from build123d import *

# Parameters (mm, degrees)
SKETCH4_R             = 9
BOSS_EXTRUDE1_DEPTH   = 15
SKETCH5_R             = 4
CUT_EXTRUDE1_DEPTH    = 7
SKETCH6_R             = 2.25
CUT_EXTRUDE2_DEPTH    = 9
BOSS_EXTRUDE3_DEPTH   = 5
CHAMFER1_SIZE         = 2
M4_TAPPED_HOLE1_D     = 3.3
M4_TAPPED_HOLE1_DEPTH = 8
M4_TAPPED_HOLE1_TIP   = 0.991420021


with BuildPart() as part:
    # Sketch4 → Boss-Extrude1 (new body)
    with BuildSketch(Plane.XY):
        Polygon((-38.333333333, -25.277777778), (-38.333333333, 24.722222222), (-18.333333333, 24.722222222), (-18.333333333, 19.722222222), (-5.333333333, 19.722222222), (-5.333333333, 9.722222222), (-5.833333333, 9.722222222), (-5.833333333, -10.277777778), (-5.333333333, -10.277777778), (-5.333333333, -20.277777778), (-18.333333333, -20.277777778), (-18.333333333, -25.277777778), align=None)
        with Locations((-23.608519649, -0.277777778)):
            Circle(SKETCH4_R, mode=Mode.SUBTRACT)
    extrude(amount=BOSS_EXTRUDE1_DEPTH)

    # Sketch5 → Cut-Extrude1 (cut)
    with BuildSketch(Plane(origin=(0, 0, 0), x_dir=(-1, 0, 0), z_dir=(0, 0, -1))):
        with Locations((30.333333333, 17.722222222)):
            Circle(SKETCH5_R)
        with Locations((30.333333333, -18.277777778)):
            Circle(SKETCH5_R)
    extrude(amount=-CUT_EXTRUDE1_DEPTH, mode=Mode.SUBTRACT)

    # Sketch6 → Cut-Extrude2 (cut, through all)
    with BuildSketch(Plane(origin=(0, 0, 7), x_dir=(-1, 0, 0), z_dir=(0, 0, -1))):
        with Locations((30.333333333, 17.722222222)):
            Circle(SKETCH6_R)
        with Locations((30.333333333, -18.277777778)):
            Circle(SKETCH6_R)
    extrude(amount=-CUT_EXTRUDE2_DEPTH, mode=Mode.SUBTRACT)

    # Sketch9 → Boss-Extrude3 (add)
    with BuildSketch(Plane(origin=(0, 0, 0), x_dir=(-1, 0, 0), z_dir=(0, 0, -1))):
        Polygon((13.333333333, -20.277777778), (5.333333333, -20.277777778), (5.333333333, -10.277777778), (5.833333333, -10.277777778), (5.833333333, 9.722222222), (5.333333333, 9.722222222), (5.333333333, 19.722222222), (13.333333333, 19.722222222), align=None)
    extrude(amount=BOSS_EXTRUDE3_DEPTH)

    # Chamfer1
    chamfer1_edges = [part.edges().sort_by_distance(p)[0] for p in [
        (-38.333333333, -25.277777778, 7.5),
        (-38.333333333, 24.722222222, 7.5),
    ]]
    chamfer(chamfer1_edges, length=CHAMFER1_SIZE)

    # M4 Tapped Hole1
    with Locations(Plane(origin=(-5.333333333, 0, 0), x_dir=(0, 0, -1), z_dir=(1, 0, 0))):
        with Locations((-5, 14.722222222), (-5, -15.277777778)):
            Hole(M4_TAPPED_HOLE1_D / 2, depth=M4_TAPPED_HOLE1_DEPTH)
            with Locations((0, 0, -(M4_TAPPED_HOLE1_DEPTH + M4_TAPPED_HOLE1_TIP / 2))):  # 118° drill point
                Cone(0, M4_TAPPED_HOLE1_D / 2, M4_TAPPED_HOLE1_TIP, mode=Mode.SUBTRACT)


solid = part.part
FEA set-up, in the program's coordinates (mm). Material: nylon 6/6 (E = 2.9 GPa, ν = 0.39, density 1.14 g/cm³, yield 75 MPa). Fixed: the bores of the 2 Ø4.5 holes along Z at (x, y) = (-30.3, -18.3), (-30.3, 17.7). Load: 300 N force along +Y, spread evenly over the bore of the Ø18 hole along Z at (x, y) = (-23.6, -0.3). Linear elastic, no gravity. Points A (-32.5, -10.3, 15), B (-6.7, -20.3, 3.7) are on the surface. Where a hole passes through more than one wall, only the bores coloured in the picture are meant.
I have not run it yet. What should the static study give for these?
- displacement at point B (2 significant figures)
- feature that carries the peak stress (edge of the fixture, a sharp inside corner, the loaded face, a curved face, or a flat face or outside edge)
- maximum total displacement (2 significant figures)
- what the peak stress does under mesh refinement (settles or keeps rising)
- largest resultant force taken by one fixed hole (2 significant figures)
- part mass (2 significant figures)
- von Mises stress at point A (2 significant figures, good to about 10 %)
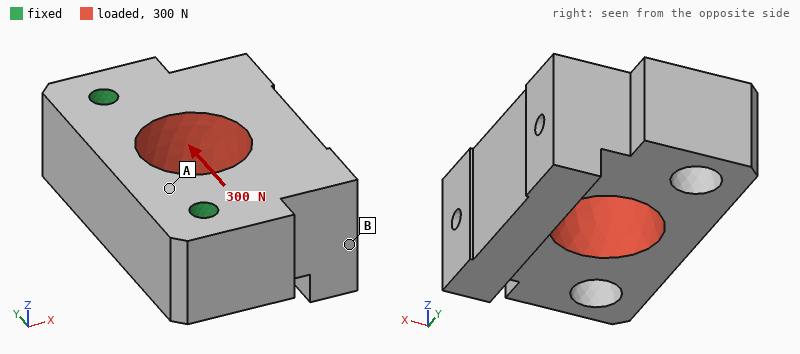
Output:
13 µm
edge of the fixture
14 µm
keeps rising
160 N
22 g
0.84 MPa
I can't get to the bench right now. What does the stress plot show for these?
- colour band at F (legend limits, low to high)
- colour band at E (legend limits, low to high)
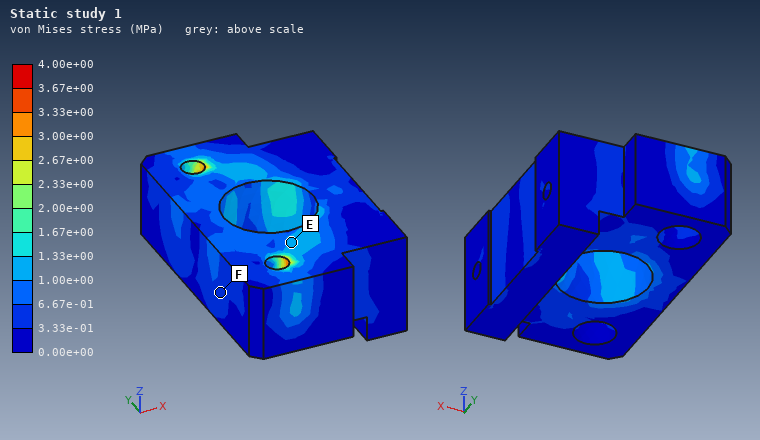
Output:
3.33e-01 to 6.67e-01 MPa
1.00e+00 to 1.33e+00 MPa
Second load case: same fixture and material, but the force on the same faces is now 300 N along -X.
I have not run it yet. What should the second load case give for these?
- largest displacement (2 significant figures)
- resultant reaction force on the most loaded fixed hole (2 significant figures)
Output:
30 µm
150 N
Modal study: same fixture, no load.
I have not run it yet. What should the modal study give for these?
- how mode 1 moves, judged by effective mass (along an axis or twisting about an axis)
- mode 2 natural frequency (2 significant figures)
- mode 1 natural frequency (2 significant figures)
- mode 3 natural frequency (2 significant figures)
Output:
along Z
4900 Hz
2300 Hz
5000 Hz
